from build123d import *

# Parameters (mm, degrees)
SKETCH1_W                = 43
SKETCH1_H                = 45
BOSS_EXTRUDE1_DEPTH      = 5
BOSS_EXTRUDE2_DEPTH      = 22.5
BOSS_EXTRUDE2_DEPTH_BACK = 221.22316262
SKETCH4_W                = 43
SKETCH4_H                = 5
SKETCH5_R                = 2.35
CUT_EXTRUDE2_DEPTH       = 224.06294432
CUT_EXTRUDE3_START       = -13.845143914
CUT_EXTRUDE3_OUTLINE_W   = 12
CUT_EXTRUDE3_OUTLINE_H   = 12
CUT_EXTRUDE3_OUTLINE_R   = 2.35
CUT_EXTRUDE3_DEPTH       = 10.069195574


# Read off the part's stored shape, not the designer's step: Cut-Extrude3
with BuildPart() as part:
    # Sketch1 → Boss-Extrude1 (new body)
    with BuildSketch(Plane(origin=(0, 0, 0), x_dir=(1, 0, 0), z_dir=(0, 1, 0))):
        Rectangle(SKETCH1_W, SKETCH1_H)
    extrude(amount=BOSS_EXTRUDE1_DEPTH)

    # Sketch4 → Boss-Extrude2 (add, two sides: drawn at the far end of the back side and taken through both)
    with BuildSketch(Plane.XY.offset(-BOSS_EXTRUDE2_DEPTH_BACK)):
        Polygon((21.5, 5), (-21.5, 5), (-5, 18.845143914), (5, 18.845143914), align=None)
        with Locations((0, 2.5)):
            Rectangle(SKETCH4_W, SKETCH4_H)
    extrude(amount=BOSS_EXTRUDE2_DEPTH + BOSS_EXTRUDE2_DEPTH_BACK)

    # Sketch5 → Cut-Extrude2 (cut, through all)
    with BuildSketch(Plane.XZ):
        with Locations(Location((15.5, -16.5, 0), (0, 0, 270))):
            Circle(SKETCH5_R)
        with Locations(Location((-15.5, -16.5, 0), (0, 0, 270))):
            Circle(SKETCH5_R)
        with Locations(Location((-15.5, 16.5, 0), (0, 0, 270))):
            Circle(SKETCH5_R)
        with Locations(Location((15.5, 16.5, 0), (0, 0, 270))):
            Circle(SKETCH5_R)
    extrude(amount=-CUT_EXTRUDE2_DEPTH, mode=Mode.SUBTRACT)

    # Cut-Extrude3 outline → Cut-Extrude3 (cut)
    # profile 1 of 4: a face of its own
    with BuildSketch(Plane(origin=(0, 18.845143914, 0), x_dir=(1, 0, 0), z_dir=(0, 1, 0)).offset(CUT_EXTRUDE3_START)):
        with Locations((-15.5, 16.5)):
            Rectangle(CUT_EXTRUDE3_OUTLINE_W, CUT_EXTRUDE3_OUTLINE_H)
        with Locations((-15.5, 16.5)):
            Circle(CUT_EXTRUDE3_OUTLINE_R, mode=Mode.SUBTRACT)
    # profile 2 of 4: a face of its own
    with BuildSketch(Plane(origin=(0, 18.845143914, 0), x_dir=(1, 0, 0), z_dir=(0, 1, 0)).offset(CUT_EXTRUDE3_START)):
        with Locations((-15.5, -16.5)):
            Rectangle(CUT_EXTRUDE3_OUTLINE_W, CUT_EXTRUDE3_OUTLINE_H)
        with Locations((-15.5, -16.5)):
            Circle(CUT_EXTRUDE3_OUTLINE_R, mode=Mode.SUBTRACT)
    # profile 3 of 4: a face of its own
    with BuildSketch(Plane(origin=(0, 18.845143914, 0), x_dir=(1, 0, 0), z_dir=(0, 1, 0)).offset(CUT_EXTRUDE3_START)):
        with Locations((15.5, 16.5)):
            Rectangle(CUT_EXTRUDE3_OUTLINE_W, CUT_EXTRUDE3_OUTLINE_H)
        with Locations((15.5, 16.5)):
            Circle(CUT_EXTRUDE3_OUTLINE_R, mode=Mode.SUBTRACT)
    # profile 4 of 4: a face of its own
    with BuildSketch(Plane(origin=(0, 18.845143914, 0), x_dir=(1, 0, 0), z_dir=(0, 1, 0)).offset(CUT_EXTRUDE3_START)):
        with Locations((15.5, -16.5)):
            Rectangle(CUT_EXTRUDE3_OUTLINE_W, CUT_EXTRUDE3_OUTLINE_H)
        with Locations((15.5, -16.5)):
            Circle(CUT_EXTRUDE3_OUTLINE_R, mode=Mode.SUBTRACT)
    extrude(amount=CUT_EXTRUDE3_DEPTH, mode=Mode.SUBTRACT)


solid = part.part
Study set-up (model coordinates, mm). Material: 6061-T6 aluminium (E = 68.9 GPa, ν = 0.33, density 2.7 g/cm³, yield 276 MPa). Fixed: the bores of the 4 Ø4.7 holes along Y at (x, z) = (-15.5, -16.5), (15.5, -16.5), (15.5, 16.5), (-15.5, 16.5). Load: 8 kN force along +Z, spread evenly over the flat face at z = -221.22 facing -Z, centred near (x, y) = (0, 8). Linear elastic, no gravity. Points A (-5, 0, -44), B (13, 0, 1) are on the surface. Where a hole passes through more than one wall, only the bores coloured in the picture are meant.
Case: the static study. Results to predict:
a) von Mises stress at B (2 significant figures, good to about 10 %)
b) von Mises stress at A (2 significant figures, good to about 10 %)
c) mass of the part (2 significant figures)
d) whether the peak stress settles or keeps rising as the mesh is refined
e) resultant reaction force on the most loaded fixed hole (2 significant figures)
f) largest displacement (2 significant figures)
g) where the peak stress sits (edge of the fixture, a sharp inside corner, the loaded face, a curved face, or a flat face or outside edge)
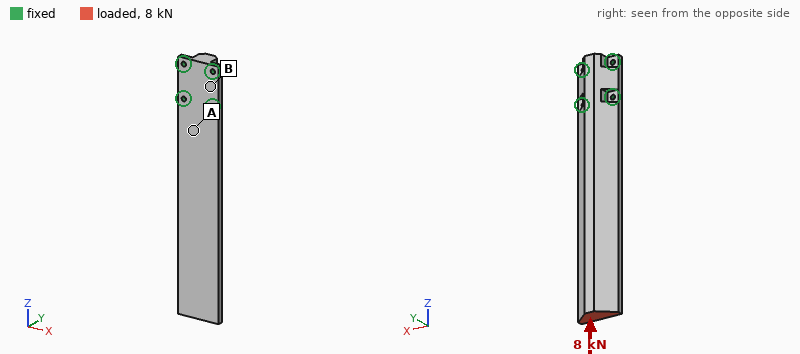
5.1 MPa
13 MPa
370 g
keeps rising
2.9 kN
0.14 mm
edge of the fixture
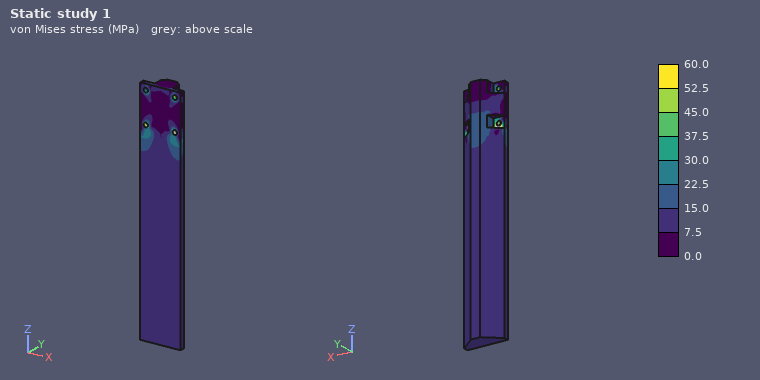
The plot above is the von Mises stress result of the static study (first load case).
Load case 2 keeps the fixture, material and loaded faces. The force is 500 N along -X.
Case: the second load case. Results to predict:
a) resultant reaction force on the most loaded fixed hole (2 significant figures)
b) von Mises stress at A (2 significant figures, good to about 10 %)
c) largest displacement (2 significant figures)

2.8 kN
8.6 MPa
0.38 mm
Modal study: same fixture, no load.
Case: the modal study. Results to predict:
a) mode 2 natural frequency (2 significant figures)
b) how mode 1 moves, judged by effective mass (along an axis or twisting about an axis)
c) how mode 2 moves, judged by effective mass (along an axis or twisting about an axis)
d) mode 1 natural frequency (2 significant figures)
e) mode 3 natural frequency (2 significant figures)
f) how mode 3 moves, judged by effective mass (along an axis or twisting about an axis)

640 Hz
along Y
along X
290 Hz
1800 Hz
along Y
